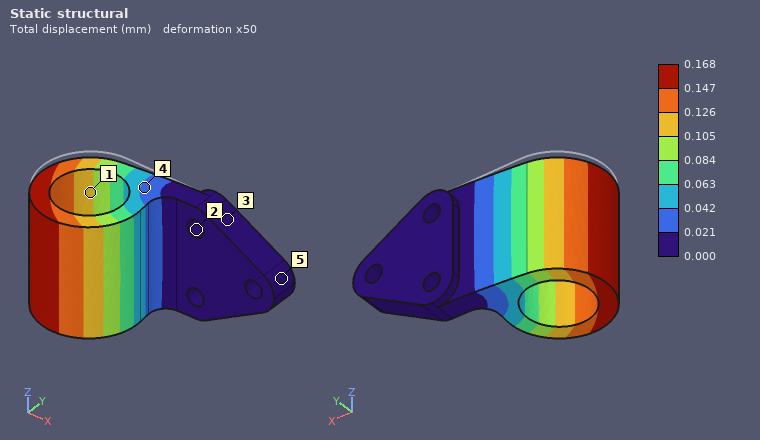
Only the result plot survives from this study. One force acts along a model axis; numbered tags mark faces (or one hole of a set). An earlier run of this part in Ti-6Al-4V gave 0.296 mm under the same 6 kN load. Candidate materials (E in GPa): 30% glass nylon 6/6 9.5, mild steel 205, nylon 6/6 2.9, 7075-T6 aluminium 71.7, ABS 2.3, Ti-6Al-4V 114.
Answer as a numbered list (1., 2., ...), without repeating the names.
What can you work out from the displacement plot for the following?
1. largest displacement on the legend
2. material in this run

1. 0.168 mm
2. mild steel
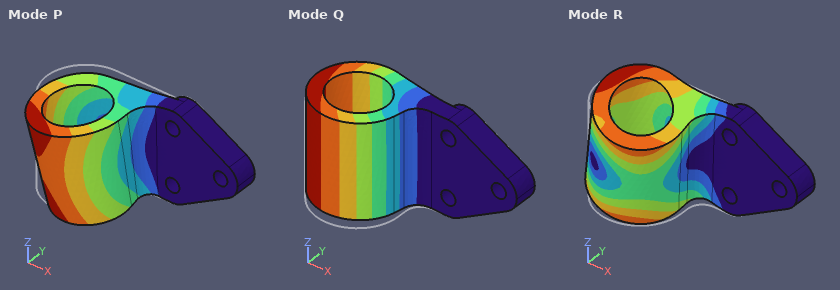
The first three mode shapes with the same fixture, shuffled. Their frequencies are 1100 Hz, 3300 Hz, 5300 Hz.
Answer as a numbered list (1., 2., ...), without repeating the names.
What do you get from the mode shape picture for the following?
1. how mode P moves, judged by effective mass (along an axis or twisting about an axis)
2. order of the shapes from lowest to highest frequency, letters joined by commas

1. along Z
2. Q, P, R
